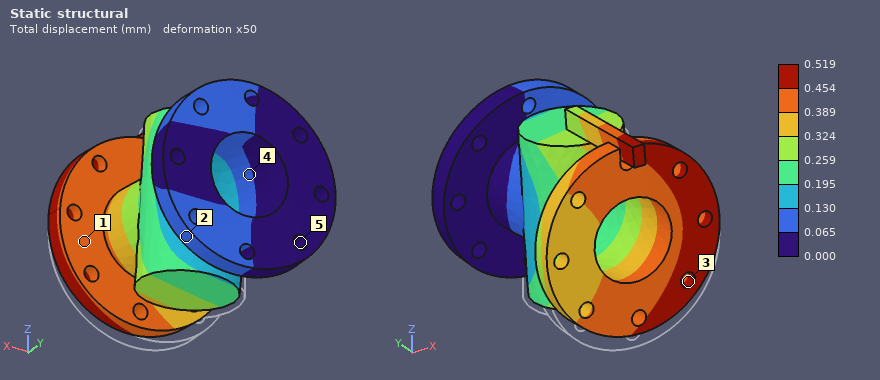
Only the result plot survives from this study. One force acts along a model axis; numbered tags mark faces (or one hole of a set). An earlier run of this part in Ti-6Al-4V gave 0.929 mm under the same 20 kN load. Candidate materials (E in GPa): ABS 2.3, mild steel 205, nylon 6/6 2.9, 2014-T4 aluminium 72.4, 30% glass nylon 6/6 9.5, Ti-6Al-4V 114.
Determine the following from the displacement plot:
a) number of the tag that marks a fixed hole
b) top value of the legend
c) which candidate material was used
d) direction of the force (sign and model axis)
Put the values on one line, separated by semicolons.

5; 0.519 mm; mild steel; +Z
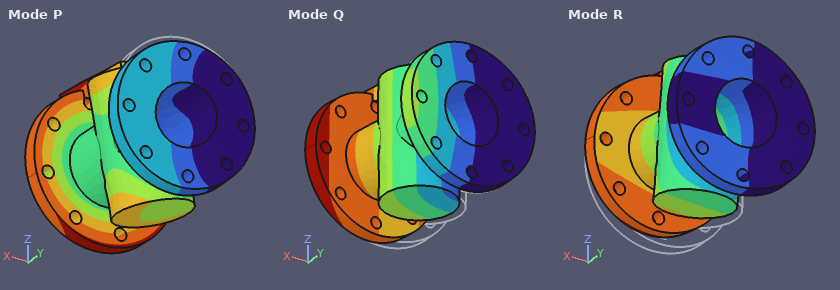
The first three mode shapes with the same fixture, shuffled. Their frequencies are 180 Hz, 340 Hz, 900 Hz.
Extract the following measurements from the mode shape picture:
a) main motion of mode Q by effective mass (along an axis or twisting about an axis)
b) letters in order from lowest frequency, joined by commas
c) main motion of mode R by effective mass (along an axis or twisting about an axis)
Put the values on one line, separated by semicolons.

along X; Q, R, P; along Z
